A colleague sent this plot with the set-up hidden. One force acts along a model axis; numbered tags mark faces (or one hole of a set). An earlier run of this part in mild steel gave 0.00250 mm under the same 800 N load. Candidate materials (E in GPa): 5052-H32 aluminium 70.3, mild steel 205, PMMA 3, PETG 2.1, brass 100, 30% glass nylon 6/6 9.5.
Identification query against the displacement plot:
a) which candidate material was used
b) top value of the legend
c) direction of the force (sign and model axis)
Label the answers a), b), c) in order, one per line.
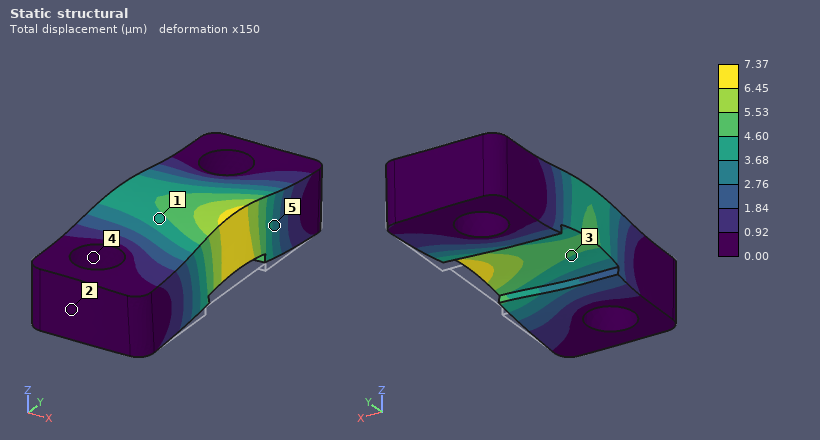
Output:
a) 5052-H32 aluminium
b) 7.37 µm
c) +Z
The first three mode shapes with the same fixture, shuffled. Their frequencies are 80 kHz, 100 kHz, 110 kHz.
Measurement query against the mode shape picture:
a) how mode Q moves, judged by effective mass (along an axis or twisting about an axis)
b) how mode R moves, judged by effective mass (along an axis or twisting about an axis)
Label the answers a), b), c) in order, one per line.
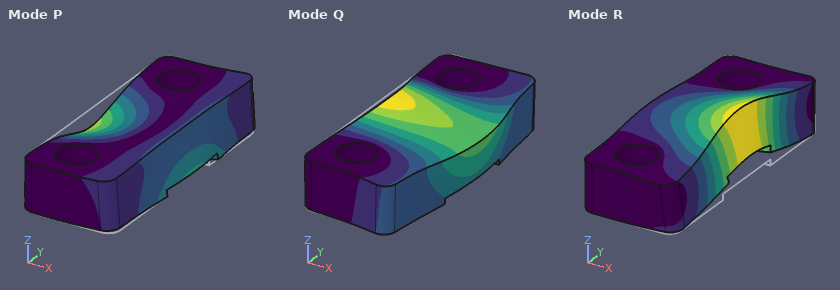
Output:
a) along X
b) along Z
